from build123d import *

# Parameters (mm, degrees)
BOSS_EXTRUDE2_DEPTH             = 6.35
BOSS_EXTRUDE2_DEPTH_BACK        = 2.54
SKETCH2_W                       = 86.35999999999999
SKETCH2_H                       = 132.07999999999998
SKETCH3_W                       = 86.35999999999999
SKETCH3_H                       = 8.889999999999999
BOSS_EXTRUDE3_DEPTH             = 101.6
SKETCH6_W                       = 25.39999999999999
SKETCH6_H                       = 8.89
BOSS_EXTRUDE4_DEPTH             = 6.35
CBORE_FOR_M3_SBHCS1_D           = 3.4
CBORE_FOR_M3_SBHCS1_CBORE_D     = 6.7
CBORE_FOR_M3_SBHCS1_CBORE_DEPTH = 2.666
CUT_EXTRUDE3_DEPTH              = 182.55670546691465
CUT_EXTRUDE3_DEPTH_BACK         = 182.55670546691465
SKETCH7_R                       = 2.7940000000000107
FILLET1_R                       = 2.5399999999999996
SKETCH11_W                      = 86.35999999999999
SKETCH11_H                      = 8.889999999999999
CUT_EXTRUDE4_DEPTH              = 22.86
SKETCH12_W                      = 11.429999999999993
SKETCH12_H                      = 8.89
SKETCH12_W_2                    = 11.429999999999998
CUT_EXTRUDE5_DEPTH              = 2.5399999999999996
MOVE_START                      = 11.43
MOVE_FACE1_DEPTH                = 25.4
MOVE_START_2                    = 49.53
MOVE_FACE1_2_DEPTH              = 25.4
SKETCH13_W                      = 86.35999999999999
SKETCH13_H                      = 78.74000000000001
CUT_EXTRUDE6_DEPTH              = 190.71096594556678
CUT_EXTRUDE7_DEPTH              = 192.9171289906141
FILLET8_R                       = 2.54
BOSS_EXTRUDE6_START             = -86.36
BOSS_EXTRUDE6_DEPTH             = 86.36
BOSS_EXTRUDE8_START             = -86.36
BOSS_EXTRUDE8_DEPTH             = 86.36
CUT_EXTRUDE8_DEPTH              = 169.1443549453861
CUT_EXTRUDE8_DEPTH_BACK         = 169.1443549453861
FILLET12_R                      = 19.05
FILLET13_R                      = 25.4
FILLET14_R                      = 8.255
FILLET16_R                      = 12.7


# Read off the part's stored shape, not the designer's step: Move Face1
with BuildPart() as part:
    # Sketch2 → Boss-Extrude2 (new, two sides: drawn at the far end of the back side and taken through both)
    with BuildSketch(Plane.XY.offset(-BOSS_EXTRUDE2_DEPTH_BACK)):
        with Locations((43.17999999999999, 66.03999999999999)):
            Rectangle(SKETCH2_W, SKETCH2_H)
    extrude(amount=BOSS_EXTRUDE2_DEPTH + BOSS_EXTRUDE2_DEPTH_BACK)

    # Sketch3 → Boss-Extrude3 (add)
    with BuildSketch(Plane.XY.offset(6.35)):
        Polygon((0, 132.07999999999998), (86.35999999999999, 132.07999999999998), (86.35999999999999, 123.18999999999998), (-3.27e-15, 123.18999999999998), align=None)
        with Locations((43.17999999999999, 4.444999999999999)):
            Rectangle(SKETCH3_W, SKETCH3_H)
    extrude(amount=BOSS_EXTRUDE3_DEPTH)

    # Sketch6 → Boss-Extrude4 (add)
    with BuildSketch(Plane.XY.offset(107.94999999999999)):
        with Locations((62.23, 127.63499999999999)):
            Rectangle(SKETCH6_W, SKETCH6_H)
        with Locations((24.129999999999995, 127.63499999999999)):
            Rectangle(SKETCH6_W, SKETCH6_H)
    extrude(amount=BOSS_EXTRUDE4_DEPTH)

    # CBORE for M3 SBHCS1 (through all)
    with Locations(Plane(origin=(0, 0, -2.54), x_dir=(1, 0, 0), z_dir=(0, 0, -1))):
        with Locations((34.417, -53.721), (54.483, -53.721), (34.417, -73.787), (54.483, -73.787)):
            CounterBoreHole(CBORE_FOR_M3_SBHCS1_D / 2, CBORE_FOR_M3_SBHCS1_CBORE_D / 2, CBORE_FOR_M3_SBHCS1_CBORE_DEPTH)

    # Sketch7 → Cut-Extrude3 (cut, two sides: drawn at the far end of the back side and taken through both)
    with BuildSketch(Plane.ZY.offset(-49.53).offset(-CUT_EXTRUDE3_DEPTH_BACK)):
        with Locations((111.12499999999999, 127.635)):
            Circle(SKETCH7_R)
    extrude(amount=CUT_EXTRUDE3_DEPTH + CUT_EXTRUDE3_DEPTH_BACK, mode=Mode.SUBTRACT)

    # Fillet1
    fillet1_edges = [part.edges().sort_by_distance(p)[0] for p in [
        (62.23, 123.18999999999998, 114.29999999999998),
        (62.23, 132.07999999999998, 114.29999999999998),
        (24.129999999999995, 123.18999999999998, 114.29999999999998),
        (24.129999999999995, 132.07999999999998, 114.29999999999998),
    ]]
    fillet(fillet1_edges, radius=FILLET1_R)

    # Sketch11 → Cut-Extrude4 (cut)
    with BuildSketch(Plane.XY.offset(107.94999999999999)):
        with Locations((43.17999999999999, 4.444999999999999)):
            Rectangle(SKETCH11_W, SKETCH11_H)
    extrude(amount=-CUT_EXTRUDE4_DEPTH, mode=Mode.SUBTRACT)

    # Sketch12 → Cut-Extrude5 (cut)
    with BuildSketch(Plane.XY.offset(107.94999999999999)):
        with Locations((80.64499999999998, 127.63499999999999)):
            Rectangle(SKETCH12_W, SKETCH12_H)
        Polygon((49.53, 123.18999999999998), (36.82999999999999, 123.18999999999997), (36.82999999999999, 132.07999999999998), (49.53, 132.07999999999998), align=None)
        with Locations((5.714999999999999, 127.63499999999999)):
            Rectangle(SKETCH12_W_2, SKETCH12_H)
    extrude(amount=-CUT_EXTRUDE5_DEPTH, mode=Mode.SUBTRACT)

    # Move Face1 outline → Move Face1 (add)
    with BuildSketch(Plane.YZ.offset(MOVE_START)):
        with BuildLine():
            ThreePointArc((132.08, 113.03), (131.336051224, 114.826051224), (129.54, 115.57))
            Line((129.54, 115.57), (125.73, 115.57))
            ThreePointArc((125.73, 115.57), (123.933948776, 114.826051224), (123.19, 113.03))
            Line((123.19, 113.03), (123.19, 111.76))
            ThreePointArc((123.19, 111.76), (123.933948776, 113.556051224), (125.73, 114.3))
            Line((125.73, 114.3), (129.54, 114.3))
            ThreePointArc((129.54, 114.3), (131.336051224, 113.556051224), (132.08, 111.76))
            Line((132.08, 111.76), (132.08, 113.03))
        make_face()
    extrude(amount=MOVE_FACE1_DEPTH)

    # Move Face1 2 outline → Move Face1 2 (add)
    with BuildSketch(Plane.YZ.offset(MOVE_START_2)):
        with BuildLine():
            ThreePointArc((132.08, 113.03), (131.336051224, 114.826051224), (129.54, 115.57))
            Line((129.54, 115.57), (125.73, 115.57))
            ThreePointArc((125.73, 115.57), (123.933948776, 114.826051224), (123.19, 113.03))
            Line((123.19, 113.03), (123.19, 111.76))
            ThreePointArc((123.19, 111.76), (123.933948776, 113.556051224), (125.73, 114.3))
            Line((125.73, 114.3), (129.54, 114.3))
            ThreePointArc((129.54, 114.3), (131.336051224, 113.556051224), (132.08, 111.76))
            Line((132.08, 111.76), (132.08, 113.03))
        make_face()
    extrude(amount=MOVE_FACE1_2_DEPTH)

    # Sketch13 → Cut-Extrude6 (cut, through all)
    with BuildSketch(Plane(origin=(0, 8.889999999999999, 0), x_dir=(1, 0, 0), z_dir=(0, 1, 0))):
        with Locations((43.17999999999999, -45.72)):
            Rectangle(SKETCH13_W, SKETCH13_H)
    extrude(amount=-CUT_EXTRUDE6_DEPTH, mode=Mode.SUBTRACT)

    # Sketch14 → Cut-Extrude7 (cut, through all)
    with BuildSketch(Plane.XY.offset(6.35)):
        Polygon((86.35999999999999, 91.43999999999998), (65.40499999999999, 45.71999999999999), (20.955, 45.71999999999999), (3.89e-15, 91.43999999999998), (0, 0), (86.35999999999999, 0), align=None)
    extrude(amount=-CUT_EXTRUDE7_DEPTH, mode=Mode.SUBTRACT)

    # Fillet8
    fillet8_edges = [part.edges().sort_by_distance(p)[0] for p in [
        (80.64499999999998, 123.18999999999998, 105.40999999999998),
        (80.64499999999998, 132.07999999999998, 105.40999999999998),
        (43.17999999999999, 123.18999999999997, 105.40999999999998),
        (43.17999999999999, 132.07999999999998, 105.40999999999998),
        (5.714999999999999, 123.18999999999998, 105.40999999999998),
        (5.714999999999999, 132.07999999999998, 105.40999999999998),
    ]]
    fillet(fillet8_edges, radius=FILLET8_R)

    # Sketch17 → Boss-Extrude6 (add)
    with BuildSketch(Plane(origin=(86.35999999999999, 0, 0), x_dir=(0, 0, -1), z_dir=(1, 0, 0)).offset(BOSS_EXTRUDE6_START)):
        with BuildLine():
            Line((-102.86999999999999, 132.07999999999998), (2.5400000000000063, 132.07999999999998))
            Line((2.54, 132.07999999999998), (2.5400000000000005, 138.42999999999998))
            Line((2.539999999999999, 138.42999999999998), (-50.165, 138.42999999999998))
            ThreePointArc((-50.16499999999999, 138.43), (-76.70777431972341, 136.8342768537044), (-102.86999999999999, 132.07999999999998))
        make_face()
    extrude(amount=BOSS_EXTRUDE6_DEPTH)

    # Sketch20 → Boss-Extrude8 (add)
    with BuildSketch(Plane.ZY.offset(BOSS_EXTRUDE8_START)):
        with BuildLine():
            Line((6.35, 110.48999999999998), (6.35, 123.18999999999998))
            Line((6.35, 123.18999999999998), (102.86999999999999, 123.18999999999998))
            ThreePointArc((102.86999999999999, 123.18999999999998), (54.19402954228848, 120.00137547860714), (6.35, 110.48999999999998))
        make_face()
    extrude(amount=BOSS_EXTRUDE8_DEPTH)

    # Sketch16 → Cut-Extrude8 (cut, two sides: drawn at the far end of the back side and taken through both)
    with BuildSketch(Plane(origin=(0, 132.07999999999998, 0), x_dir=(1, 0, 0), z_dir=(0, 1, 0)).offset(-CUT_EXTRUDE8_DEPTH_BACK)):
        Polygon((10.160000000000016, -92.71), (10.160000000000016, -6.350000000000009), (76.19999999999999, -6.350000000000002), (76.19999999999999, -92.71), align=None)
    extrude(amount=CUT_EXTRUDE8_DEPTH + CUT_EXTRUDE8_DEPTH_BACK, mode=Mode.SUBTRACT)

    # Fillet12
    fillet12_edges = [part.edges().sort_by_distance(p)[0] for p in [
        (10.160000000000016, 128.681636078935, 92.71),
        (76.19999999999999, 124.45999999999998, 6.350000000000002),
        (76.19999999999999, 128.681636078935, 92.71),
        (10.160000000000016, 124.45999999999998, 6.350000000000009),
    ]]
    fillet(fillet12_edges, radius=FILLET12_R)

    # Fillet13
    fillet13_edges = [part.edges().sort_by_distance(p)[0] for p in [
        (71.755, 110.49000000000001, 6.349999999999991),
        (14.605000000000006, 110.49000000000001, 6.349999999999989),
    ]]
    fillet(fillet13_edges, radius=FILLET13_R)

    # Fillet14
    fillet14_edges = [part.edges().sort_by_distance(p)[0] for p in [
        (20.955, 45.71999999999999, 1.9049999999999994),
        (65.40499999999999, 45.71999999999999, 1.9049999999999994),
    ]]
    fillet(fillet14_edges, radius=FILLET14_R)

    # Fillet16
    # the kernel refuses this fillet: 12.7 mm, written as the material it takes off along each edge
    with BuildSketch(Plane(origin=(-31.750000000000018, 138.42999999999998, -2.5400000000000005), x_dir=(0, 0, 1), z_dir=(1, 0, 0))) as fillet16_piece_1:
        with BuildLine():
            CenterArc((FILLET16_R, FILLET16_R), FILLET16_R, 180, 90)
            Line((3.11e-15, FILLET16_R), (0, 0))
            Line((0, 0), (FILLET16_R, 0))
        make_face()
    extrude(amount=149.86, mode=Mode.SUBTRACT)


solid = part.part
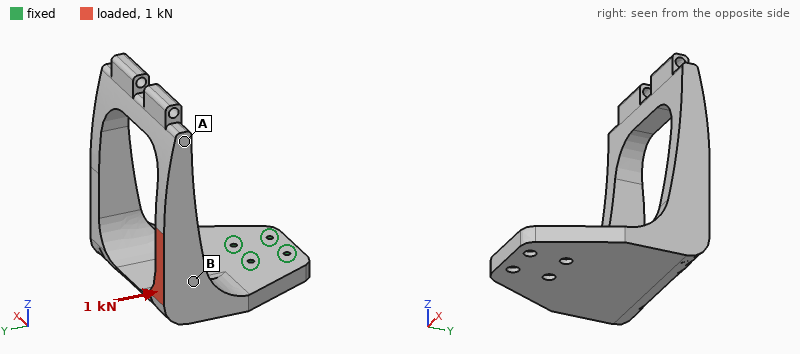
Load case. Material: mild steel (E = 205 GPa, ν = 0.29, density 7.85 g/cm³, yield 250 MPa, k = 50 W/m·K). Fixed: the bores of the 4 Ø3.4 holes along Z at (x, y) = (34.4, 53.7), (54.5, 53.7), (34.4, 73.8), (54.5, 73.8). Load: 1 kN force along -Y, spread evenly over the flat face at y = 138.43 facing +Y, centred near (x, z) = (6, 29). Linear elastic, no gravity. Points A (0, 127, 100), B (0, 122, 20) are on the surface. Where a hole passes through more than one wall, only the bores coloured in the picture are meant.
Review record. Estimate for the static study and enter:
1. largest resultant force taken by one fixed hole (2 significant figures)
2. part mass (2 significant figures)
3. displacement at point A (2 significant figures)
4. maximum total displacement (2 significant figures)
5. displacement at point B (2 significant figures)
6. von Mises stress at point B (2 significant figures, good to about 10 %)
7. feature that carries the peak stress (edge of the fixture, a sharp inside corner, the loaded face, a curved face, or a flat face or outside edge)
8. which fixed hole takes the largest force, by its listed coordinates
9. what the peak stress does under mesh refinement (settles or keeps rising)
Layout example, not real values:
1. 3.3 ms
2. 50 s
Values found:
1. 1.4 kN
2. 910 g
3. 0.15 mm
4. 0.16 mm
5. 0.055 mm
6. 7.9 MPa
7. edge of the fixture
8. (34.4, 73.8)
9. keeps rising
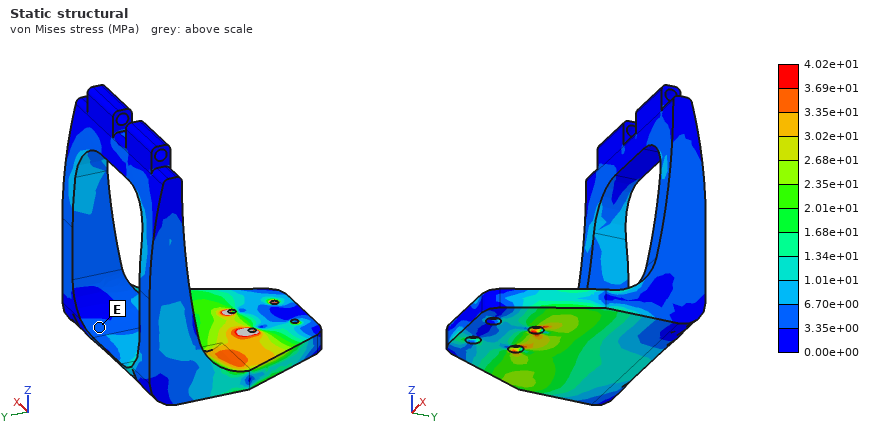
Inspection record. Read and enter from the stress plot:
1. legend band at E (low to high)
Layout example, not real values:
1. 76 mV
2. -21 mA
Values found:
1. 3.35e+00 to 6.70e+00 MPa
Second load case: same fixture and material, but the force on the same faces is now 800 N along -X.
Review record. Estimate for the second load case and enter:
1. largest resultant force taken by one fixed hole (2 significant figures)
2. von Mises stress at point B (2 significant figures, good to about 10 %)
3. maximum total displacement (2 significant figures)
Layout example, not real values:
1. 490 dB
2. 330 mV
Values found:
1. 1.5 kN
2. 9.0 MPa
3. 74 µm
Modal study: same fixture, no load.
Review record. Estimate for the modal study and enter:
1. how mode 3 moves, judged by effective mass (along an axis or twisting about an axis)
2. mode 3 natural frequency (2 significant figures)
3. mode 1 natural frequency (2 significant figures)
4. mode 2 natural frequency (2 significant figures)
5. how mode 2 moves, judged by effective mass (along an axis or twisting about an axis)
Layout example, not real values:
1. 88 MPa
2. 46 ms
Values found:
1. along Z
2. 1600 Hz
3. 450 Hz
4. 590 Hz
5. along X
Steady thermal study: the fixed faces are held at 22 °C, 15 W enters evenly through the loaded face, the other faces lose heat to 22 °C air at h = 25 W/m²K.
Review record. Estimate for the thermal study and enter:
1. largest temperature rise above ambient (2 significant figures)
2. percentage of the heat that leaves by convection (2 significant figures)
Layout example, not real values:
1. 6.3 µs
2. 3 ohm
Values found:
1. 36 K
2. 53 %
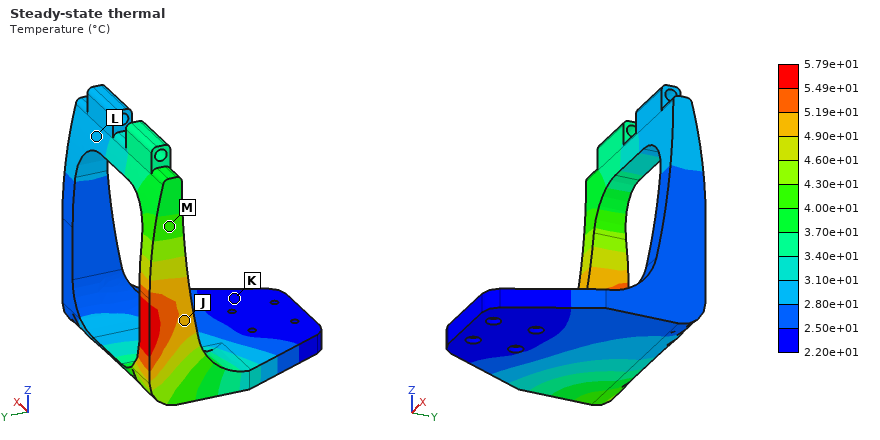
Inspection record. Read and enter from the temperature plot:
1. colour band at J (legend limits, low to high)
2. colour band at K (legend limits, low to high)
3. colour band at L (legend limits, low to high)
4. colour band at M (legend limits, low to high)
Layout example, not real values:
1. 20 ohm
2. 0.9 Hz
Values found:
1. 4.90e+01 to 5.19e+01 °C
2. 2.20e+01 to 2.50e+01 °C
3. 2.80e+01 to 3.10e+01 °C
4. 4.00e+01 to 4.30e+01 °C
